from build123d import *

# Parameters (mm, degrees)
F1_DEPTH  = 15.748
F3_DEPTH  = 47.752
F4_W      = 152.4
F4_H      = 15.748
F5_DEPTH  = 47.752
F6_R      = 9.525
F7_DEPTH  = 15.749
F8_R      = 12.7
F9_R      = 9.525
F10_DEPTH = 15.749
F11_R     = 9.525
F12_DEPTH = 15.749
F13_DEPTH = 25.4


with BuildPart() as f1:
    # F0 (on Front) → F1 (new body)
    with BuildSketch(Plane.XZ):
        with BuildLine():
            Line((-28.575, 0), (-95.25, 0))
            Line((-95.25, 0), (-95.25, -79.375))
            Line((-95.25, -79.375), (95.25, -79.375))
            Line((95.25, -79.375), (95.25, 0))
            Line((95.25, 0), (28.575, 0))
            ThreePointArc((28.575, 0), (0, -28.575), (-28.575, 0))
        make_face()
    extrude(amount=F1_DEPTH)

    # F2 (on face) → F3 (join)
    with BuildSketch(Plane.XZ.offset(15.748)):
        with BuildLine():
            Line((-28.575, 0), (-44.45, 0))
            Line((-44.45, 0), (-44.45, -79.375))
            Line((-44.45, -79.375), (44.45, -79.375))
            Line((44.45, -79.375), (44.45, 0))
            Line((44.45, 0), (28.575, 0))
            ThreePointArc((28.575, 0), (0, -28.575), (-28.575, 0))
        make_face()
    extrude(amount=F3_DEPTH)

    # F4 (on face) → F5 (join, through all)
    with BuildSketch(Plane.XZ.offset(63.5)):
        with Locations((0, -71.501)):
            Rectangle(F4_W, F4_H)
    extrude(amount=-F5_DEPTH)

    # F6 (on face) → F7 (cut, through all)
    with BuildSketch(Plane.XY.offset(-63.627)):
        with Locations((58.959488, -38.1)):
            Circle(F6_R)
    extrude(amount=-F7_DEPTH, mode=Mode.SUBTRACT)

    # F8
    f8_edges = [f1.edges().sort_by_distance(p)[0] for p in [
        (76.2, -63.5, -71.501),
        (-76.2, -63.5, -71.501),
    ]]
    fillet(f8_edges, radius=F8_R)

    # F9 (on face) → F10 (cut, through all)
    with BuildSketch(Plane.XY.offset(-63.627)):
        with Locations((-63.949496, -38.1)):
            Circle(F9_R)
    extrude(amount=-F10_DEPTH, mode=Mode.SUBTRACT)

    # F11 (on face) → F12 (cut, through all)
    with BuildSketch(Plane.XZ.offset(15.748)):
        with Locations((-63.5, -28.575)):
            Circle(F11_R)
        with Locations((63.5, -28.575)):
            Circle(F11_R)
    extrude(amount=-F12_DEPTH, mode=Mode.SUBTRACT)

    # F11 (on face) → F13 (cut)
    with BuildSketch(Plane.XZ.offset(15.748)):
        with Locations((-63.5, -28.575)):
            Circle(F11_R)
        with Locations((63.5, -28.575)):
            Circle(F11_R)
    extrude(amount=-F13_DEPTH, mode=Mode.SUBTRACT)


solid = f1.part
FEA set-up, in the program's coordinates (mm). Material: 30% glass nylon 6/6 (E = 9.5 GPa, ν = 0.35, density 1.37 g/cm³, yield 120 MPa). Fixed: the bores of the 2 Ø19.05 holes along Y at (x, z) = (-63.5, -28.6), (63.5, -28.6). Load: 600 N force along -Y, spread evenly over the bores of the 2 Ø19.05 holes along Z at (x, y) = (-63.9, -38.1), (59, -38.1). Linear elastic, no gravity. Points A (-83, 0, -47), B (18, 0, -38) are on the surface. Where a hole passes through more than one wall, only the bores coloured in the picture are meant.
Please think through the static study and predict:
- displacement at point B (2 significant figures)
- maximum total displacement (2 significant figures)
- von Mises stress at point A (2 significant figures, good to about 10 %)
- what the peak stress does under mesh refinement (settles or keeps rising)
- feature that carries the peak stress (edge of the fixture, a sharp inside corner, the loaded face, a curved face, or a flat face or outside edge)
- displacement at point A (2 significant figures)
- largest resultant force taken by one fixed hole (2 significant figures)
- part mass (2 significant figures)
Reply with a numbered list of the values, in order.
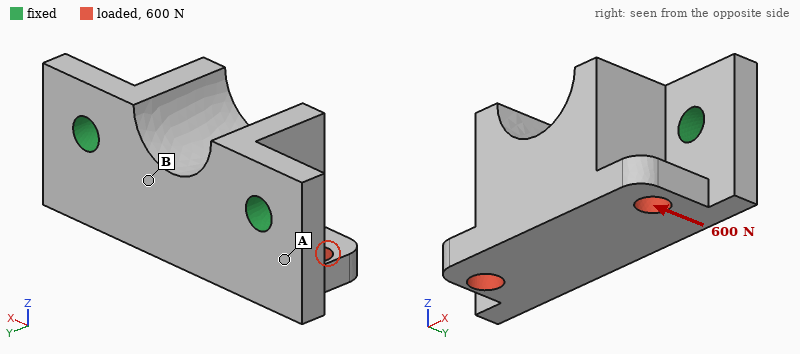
1. 7.4 µm
2. 41 µm
3. 1.3 MPa
4. keeps rising
5. edge of the fixture
6. 6.9 µm
7. 310 N
8. 720 g
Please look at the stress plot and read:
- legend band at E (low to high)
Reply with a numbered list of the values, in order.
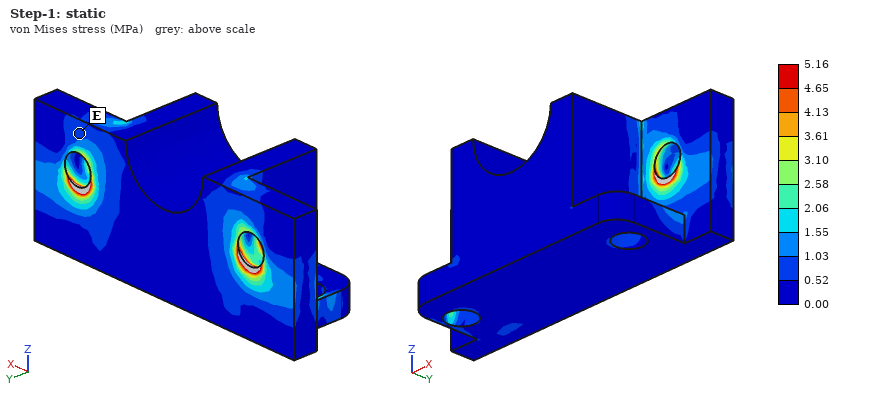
1. 0.52 to 1.03 MPa
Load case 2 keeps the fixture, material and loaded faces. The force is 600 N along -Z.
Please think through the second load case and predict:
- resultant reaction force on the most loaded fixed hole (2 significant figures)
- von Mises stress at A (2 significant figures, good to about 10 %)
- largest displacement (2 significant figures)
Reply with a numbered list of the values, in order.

1. 320 N
2. 1.0 MPa
3. 47 µm
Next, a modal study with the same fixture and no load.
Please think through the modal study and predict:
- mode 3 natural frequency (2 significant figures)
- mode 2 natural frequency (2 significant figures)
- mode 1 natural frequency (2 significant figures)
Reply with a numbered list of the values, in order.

1. 2600 Hz
2. 2600 Hz
3. 1000 Hz
